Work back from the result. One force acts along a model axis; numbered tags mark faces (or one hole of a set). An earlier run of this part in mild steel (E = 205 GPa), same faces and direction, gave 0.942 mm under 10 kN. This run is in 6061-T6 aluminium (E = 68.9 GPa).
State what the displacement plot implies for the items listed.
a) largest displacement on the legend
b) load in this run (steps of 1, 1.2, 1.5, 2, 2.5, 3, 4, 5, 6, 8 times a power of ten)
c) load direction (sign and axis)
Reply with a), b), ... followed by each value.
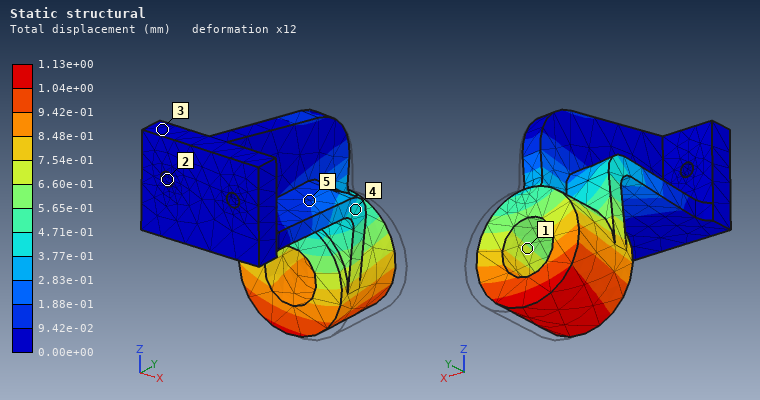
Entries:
a) 1.13e+00 mm
b) 4 kN
c) -X
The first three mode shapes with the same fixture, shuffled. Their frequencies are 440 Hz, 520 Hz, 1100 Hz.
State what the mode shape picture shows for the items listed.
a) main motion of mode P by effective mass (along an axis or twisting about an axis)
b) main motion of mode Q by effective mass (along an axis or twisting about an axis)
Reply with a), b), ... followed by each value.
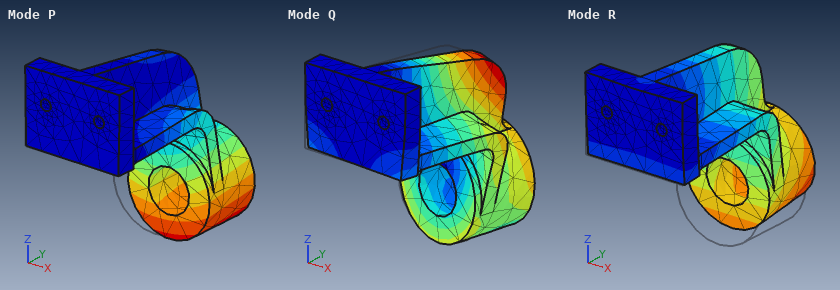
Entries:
a) along X
b) along X
